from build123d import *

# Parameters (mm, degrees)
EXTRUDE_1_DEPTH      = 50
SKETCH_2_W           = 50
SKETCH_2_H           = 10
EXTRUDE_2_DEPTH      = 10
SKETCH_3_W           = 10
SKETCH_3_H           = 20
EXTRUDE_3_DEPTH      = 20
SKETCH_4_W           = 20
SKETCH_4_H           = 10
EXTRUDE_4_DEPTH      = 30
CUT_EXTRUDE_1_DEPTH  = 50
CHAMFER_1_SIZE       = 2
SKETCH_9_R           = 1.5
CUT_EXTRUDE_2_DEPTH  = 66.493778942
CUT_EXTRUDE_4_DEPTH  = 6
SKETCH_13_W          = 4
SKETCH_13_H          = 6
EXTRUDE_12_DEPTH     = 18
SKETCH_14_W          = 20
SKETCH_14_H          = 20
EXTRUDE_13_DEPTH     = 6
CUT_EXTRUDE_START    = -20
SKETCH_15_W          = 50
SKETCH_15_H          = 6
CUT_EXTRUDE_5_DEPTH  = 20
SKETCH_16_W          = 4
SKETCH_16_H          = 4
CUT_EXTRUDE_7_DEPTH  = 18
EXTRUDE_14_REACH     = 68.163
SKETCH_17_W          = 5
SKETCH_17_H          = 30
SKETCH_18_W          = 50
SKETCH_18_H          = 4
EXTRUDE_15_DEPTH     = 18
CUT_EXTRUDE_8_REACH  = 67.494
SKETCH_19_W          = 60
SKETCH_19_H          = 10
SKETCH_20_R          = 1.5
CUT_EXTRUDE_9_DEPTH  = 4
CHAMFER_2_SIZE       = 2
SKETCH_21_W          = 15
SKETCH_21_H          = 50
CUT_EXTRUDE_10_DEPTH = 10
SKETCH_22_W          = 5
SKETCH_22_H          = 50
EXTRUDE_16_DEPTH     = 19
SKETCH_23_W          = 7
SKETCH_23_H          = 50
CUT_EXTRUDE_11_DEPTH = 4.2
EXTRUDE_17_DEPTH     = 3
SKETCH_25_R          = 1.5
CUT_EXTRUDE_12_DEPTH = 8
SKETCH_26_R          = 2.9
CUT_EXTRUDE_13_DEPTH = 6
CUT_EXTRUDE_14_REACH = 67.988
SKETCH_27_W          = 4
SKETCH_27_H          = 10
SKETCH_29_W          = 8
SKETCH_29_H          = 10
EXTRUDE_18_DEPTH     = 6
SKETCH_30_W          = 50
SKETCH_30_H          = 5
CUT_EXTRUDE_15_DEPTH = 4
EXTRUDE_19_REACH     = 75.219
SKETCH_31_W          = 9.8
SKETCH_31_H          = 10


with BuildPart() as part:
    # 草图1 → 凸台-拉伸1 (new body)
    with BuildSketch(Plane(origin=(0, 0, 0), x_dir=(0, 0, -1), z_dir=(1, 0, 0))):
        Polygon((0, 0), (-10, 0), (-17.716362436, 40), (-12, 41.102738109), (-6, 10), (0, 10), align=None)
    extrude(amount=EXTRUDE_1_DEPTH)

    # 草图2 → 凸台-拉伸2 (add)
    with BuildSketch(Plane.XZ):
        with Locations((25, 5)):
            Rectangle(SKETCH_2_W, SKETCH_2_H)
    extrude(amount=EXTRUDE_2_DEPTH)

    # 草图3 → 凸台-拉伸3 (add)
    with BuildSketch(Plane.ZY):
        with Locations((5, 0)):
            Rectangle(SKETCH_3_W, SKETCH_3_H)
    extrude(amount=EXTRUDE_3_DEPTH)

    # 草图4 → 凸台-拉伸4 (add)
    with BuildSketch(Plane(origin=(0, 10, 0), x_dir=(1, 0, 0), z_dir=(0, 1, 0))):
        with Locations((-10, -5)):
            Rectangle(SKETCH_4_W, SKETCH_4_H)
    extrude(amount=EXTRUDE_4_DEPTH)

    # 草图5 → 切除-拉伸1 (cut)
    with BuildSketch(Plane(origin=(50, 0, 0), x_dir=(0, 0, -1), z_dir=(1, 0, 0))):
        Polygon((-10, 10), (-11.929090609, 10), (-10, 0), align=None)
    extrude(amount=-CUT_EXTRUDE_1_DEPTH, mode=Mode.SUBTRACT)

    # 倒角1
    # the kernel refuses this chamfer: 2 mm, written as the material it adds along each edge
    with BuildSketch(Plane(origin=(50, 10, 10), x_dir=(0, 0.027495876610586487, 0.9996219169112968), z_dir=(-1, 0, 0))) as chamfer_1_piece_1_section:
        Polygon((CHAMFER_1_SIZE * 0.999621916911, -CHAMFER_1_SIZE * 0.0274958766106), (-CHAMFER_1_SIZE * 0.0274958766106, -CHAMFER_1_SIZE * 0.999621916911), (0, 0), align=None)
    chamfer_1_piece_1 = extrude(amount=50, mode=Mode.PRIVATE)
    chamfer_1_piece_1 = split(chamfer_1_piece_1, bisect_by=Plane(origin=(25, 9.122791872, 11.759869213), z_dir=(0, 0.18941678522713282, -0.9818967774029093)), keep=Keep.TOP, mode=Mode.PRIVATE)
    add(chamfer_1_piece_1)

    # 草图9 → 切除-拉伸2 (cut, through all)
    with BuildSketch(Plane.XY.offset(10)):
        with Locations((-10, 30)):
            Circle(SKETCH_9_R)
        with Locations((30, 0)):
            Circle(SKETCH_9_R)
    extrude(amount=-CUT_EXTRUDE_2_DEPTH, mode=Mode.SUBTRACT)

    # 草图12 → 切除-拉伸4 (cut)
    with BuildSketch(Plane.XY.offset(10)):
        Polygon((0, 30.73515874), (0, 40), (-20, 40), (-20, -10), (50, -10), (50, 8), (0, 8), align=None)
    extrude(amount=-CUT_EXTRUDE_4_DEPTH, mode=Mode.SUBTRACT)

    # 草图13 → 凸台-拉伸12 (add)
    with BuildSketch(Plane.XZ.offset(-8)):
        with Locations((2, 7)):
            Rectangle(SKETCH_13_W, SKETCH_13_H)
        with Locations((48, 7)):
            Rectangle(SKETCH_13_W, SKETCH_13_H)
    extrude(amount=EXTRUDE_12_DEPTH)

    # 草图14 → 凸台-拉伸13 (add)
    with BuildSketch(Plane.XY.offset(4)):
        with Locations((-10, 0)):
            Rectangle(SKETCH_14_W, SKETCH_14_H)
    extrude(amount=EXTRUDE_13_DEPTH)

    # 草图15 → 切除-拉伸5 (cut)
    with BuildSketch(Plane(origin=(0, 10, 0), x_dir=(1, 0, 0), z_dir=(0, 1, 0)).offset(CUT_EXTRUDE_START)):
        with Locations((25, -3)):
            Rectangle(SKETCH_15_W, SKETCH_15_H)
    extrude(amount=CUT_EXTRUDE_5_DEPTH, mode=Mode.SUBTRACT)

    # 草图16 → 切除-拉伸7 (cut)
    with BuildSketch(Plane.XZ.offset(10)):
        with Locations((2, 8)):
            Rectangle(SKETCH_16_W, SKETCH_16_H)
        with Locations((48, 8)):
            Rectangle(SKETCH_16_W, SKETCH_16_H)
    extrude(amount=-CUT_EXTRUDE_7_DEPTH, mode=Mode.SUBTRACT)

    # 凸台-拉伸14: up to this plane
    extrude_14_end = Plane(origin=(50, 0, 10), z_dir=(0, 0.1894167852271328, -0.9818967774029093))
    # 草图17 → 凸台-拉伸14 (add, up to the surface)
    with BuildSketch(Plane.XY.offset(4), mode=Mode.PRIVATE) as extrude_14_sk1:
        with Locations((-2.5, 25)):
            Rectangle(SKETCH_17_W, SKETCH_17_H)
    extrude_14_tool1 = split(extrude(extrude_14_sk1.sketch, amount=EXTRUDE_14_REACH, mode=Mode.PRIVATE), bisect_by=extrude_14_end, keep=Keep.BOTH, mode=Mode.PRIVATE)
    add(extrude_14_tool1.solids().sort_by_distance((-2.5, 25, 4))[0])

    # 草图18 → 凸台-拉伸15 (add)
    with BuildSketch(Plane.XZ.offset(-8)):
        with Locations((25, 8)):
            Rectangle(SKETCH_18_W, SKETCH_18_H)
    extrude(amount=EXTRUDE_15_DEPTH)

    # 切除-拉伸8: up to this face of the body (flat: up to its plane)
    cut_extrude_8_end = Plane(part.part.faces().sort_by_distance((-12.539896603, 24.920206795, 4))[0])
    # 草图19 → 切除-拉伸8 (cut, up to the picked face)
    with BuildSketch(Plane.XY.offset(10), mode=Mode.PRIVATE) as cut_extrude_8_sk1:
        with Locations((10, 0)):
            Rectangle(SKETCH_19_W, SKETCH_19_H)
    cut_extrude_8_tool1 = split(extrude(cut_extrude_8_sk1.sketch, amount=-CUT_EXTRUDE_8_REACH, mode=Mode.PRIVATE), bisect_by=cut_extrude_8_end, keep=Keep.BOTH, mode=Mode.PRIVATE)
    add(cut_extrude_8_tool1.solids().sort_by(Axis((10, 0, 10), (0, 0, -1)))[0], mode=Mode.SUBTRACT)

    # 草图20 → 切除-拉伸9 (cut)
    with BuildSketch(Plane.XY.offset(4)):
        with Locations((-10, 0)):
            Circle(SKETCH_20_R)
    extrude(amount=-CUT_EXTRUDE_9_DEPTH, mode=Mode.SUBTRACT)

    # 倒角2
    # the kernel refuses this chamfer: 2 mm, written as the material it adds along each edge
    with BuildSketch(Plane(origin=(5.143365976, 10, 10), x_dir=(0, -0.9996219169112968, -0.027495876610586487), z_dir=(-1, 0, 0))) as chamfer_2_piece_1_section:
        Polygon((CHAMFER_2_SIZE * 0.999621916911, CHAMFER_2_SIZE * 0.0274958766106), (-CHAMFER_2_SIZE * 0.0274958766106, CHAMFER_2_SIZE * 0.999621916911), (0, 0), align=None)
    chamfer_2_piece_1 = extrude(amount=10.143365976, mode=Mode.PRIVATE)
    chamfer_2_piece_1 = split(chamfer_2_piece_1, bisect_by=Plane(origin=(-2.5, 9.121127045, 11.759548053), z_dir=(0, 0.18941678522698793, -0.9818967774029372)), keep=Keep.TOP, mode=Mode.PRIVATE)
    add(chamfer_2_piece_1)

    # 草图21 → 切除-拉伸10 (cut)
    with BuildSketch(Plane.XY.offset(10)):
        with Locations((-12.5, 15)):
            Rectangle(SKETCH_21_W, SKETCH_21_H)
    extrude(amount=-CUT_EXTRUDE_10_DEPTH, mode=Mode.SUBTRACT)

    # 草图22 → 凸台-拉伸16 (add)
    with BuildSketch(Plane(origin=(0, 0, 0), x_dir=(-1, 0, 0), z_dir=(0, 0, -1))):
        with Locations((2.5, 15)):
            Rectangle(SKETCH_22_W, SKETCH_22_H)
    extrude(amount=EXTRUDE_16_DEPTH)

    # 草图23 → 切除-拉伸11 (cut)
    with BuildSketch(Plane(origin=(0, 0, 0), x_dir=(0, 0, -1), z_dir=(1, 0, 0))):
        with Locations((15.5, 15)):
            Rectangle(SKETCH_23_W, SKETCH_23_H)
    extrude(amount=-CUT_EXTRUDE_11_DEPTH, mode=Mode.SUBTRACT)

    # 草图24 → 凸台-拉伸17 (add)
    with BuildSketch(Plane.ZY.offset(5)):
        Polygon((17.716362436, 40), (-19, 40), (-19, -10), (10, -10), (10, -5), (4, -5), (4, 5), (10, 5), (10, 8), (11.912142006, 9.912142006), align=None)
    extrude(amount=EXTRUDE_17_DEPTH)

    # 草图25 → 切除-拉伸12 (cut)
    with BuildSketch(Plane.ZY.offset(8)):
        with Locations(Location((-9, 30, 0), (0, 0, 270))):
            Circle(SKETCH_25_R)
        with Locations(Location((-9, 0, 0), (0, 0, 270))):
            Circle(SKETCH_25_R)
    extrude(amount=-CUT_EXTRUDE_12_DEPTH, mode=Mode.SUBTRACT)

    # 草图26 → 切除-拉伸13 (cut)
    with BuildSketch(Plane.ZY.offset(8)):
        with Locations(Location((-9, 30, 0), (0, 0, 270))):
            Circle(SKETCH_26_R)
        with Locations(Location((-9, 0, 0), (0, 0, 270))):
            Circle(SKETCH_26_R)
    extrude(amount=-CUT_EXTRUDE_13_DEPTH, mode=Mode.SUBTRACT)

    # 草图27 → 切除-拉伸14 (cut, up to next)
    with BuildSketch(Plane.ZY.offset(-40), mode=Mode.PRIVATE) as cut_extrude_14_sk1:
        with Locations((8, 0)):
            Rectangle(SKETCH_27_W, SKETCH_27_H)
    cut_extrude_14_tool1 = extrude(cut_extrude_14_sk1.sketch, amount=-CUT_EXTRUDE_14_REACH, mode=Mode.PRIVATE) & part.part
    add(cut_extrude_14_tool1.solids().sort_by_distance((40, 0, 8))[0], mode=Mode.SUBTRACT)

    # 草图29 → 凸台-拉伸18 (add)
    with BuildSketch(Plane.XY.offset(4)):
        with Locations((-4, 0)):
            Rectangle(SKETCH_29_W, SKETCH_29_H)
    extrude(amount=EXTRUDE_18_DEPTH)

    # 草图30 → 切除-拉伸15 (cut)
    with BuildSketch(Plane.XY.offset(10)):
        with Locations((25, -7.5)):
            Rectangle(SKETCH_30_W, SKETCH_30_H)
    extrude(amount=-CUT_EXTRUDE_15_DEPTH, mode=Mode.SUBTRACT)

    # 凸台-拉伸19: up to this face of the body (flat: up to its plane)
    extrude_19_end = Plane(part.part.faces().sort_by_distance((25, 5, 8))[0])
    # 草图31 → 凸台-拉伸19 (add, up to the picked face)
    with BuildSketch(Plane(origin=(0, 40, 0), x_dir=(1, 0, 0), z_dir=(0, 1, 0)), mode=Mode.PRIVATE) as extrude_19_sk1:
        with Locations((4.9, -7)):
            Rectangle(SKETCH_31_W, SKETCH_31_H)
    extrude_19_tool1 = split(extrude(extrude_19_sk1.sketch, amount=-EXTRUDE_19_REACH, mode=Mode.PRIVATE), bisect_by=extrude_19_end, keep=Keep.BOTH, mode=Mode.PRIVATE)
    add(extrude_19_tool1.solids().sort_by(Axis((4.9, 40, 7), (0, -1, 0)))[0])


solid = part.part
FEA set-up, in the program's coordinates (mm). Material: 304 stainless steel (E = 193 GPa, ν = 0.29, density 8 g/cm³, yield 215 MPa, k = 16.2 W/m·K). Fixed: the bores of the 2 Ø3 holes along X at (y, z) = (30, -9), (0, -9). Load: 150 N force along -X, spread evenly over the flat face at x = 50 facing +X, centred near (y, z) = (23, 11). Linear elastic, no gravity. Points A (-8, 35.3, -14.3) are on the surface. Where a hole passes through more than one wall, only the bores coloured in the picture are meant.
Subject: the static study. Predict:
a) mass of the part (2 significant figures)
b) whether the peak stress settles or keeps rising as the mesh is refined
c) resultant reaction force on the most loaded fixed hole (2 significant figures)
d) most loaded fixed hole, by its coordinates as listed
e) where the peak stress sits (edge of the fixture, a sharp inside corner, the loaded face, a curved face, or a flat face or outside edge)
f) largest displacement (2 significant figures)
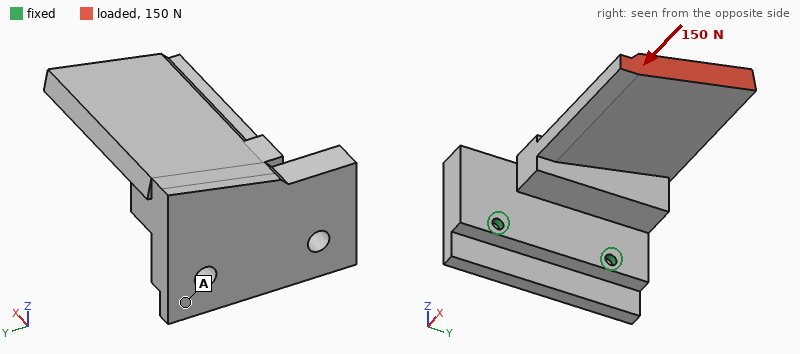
190 g
keeps rising
120 N
(30, -9)
edge of the fixture
48 µm
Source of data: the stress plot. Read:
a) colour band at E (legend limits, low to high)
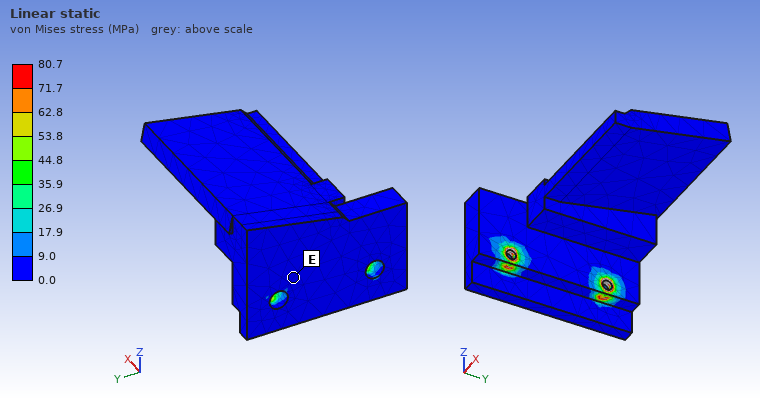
0.0 to 9.0 MPa
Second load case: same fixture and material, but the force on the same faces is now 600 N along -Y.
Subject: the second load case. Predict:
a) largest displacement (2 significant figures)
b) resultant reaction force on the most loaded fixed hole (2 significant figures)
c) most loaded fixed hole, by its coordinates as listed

66 µm
1.2 kN
(30, -9)
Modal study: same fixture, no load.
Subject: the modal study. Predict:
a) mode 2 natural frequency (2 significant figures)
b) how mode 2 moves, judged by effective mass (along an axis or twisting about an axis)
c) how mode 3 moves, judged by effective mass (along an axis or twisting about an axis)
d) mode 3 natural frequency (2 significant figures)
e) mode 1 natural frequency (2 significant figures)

2700 Hz
along Y
along X
3700 Hz
830 Hz
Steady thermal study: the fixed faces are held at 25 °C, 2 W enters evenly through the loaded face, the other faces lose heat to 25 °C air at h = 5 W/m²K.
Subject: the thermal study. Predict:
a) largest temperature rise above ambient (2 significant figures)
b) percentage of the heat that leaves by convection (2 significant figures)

34 K
28 %
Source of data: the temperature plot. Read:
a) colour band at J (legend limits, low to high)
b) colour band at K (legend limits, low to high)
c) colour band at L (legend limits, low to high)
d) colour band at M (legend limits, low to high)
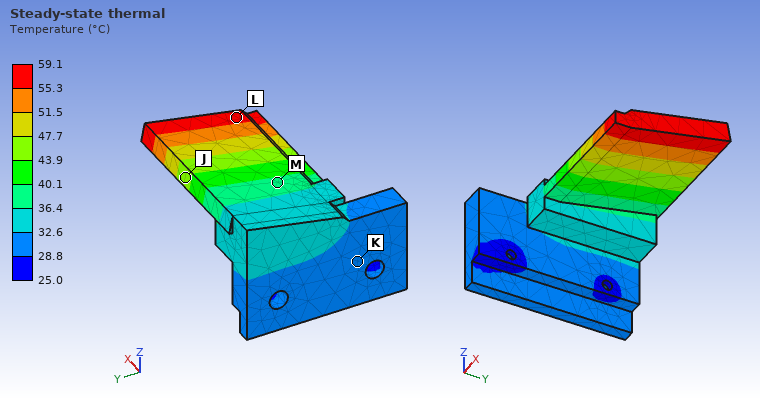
43.9 to 47.7 °C
28.8 to 32.6 °C
55.3 to 59.1 °C
36.4 to 40.1 °C
